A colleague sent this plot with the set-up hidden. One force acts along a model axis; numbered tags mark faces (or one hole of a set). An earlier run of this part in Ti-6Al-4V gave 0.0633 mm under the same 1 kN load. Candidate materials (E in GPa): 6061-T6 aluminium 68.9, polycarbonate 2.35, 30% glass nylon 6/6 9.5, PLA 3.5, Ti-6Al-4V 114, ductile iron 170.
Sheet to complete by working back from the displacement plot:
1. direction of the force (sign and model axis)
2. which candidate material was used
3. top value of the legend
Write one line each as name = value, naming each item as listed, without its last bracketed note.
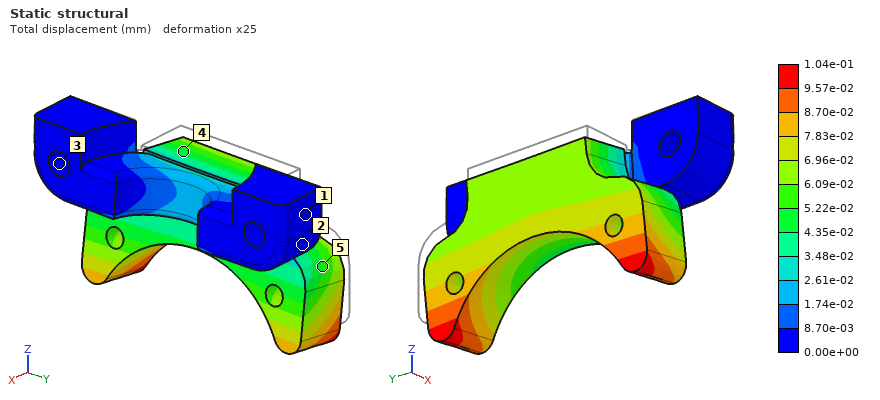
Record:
direction of the force = -Z
which candidate material was used = 6061-T6 aluminium
top value of the legend = 1.04e-01 mm
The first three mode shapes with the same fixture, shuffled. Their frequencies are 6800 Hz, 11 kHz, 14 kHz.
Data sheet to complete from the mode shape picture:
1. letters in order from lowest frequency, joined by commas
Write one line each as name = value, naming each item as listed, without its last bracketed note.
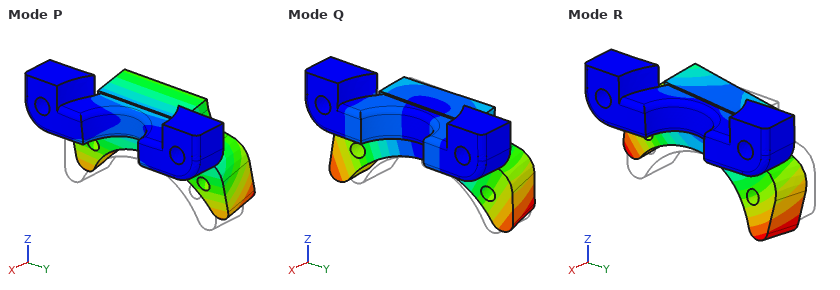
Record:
letters in order from lowest frequency, joined by commas = P, R, Q
